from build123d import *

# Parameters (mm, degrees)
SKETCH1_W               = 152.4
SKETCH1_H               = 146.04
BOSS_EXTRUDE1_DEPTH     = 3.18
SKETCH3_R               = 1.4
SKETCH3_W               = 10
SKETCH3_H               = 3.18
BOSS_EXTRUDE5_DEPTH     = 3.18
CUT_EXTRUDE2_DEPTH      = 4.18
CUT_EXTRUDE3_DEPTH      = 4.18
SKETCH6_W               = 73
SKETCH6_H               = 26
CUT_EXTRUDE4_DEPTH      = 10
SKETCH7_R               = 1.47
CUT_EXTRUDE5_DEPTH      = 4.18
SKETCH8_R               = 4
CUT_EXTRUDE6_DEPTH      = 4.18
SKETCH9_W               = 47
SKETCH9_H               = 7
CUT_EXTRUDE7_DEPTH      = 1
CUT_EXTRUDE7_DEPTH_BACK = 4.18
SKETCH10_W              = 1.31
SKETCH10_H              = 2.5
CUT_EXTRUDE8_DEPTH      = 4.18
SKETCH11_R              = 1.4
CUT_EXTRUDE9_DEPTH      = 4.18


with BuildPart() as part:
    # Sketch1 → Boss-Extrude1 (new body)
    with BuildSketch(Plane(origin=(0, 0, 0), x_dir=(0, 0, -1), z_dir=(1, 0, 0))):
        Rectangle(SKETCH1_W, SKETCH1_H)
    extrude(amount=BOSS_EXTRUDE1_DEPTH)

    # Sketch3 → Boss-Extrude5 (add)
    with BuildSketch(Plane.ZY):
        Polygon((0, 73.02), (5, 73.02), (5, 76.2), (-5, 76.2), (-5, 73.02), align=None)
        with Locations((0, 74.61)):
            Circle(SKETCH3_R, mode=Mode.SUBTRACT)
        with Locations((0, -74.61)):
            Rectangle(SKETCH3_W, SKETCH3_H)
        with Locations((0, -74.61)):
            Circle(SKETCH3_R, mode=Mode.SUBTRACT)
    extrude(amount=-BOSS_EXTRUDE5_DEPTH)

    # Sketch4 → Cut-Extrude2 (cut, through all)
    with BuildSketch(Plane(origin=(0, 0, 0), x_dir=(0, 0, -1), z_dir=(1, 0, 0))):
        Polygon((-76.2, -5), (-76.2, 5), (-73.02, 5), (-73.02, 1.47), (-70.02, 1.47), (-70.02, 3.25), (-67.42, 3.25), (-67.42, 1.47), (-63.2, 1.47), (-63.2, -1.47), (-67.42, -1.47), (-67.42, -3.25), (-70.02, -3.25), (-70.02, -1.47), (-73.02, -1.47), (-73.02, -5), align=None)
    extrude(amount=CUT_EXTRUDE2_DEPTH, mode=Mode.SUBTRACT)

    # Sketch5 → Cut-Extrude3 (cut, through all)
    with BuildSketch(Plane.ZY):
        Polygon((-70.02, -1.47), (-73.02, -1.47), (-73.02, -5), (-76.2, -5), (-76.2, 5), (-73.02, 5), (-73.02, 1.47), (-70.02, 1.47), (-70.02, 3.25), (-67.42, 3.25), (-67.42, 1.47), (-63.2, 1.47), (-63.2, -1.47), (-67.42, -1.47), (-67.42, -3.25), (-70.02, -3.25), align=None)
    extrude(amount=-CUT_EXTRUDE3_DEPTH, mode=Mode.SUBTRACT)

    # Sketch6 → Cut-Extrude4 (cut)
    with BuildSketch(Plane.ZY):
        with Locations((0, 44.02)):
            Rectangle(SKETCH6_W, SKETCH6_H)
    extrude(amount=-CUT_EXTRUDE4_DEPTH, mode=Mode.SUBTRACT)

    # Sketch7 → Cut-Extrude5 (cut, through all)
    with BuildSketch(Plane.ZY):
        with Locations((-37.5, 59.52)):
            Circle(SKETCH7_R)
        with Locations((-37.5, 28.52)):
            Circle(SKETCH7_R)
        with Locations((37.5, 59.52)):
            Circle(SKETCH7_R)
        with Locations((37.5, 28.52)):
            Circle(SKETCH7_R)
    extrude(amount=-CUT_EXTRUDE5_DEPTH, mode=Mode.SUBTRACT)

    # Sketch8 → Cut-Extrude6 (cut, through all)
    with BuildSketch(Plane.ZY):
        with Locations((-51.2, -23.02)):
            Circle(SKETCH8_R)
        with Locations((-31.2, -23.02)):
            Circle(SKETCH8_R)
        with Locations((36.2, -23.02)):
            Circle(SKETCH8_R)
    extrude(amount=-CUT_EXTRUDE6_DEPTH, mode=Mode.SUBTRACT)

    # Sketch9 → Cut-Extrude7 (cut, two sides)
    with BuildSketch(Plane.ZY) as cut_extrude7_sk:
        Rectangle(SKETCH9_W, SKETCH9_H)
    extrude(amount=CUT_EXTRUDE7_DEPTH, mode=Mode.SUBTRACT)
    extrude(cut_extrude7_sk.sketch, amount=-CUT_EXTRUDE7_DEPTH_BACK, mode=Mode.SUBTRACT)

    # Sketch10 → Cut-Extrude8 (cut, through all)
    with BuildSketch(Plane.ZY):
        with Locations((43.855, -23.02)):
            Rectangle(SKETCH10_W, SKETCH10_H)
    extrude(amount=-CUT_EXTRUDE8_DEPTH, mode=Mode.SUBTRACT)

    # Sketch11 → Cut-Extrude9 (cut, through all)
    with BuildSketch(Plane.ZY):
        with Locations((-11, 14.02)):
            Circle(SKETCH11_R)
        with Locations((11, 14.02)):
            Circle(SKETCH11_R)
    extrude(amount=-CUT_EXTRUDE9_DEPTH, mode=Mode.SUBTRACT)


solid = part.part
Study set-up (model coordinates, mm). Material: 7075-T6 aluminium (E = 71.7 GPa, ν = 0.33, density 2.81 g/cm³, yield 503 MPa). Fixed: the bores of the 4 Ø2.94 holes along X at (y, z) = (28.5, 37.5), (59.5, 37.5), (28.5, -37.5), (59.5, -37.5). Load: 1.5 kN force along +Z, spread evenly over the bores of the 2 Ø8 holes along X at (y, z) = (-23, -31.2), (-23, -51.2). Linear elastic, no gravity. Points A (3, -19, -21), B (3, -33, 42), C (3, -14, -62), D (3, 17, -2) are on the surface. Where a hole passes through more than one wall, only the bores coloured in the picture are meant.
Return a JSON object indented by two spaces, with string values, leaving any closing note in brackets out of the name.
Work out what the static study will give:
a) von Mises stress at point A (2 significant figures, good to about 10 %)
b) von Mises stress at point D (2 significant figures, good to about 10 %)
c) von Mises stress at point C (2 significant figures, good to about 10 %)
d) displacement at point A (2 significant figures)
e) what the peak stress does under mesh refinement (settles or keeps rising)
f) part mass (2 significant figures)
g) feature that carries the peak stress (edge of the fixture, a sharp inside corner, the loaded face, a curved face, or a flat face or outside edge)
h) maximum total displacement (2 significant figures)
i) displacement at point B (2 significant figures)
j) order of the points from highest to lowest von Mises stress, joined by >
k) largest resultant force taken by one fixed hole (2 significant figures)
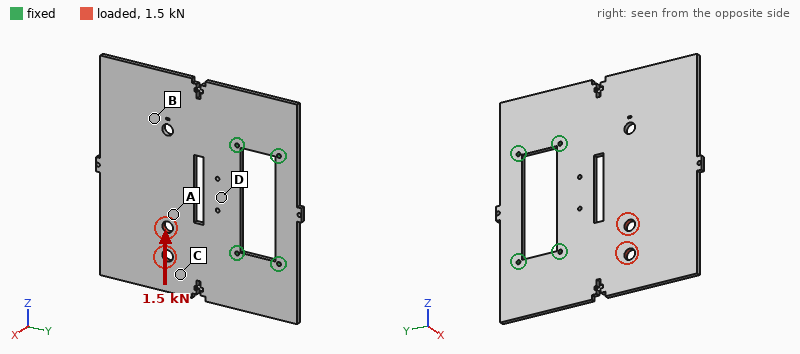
{
  "von Mises stress at point A": "13 MPa",
  "von Mises stress at point D": "9.0 MPa",
  "von Mises stress at point C": "6.4 MPa",
  "displacement at point A": "21 µm",
  "what the peak stress does under mesh refinement": "keeps rising",
  "part mass": "180 g",
  "feature that carries the peak stress": "edge of the fixture",
  "maximum total displacement": "30 µm",
  "displacement at point B": "21 µm",
  "order of the points from highest to lowest von Mises stress, joined by >": "A > D > C > B",
  "largest resultant force taken by one fixed hole": "1.2 kN"
}
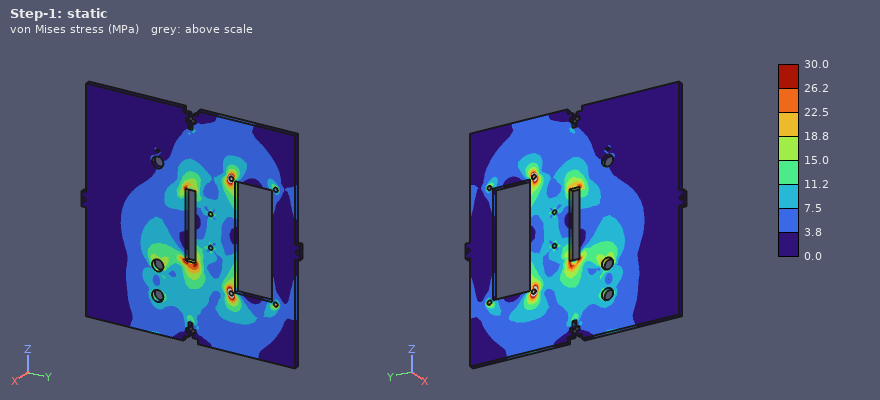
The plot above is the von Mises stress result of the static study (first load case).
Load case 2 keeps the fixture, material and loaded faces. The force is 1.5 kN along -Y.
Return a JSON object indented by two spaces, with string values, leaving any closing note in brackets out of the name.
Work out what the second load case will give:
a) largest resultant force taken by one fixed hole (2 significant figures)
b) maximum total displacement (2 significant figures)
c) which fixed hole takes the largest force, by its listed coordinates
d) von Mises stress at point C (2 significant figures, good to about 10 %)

{
  "largest resultant force taken by one fixed hole": "1.2 kN",
  "maximum total displacement": "16 µm",
  "which fixed hole takes the largest force, by its listed coordinates": "(28.5, -37.5)",
  "von Mises stress at point C": "7.5 MPa"
}
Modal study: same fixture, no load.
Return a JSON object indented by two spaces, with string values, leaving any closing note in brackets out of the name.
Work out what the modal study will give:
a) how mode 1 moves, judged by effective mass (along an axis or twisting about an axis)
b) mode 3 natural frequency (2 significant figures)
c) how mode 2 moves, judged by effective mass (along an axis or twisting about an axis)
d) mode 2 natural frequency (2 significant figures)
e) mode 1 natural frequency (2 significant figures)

{
  "how mode 1 moves, judged by effective mass": "along X",
  "mode 3 natural frequency": "880 Hz",
  "how mode 2 moves, judged by effective mass": "twisting about Y",
  "mode 2 natural frequency": "400 Hz",
  "mode 1 natural frequency": "190 Hz"
}
